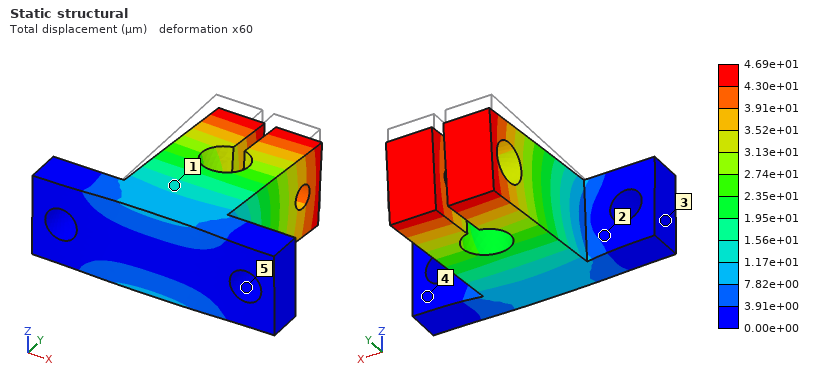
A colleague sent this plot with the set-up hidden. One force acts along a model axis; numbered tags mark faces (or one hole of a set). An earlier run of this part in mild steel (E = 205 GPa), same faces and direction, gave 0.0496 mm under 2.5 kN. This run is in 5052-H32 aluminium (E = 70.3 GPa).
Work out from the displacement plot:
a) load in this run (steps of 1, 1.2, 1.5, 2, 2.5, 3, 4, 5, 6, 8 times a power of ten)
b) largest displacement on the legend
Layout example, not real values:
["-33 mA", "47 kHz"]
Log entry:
["800 N", "4.69e+01 µm"]
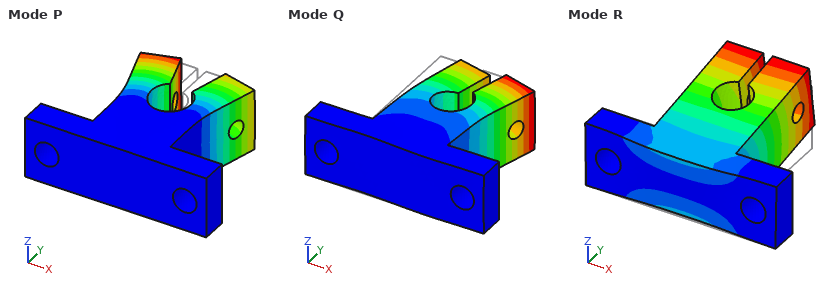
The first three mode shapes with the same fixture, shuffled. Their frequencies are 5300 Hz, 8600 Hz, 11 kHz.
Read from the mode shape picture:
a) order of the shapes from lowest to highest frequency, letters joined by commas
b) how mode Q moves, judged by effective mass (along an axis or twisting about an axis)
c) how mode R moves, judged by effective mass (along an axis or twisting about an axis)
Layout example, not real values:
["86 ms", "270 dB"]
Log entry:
["R, Q, P", "along X", "along Z"]
